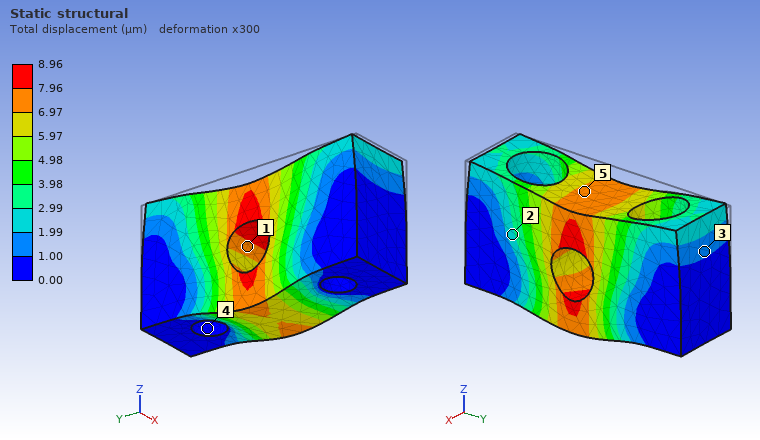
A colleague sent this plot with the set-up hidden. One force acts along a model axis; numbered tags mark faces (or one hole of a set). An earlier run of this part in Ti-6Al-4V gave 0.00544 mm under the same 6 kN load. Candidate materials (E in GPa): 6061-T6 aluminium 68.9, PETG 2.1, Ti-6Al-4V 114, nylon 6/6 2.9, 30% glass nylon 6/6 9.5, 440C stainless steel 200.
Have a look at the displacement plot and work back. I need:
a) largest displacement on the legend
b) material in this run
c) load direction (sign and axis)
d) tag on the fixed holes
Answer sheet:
8.96 µm
6061-T6 aluminium
-Z
4
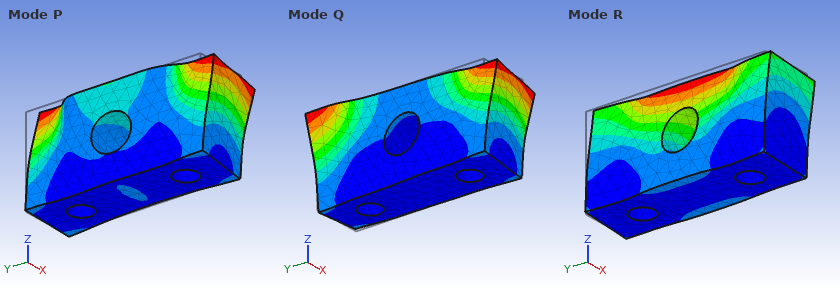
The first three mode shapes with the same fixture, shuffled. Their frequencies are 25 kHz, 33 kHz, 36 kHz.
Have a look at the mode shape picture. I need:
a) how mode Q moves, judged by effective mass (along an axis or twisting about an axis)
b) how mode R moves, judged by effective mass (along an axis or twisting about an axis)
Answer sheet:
twisting about Z
along X
